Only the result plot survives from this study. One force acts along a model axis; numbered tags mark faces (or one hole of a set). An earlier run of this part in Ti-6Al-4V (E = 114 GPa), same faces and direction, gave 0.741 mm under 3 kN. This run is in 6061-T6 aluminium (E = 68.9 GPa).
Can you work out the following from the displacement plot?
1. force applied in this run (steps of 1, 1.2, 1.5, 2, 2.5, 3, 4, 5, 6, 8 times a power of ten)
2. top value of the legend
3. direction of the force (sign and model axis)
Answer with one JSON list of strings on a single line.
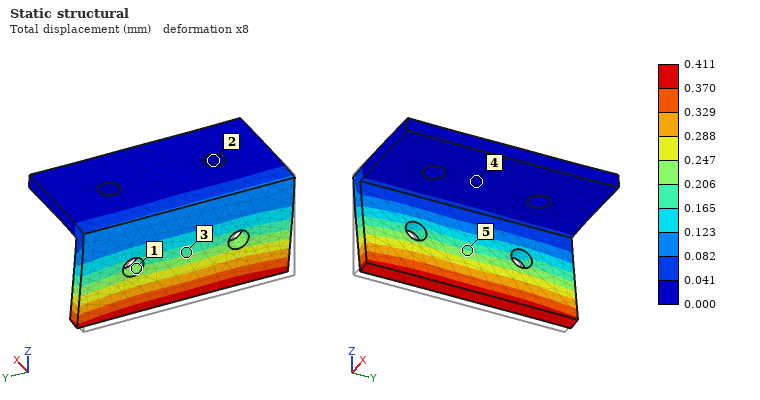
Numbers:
["1 kN", "0.411 mm", "+X"]
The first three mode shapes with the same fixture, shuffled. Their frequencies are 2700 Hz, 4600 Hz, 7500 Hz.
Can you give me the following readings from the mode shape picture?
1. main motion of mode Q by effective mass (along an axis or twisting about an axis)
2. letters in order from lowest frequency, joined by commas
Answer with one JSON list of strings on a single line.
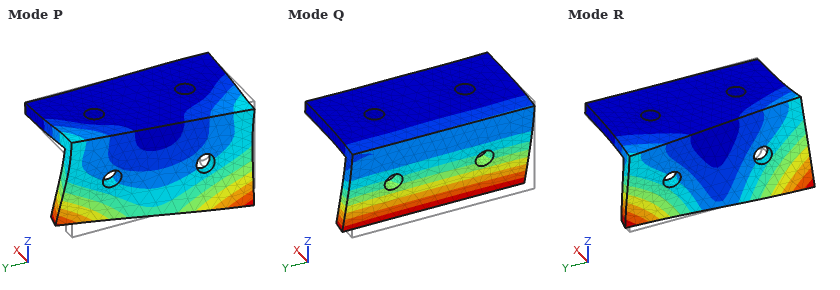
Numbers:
["along X", "Q, R, P"]
